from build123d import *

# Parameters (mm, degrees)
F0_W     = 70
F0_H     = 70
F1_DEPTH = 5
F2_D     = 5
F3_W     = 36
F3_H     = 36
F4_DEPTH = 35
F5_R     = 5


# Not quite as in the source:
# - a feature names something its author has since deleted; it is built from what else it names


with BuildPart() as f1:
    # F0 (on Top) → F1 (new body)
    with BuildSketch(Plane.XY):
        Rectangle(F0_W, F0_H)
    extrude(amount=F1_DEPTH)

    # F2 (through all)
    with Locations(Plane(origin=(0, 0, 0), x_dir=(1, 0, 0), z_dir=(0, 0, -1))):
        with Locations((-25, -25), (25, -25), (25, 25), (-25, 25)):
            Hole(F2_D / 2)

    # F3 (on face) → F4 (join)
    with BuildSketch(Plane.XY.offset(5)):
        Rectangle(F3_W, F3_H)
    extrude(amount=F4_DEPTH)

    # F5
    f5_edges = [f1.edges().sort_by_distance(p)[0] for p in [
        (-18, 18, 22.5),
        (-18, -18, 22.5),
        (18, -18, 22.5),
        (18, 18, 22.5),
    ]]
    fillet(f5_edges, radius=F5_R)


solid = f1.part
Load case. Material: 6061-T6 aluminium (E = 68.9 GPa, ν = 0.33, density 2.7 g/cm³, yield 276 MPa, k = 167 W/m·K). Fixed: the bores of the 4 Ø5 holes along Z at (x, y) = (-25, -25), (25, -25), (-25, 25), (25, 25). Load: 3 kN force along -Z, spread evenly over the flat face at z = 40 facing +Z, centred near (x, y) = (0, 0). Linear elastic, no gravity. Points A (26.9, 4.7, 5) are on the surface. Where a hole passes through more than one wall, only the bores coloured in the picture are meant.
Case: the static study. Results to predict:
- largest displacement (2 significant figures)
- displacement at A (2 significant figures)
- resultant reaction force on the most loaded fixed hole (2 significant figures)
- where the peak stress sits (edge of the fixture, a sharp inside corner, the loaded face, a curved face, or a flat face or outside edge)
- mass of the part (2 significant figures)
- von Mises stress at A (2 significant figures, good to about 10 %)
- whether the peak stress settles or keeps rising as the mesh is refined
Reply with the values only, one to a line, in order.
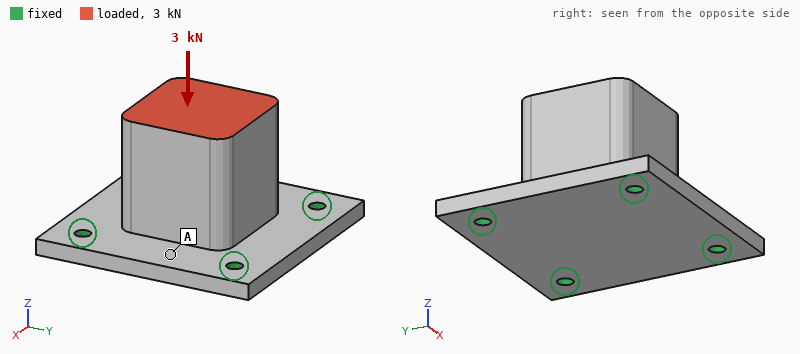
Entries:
21 µm
14 µm
800 N
edge of the fixture
190 g
11 MPa
keeps rising
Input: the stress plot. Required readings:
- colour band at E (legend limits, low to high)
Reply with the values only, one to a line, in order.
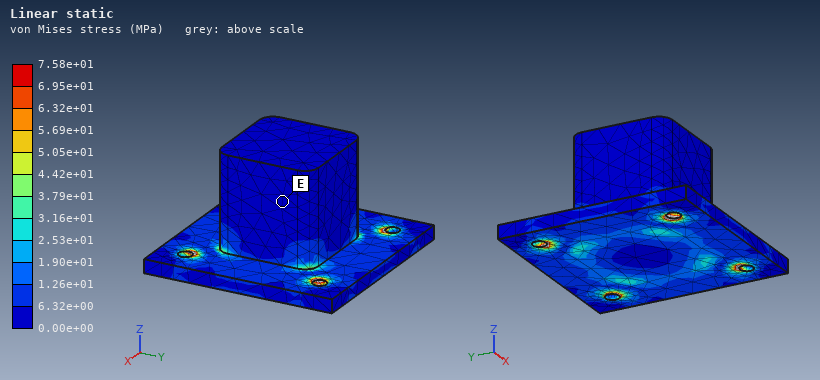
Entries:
0.00e+00 to 6.32e+00 MPa
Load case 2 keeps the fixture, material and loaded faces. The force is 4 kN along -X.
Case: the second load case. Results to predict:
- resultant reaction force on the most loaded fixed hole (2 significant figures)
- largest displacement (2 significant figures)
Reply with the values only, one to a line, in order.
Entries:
2.1 kN
0.10 mm
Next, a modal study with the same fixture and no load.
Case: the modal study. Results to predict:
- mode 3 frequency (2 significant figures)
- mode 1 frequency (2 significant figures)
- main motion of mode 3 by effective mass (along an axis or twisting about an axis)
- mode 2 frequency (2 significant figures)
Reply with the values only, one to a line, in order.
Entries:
5000 Hz
4400 Hz
along Z
4400 Hz
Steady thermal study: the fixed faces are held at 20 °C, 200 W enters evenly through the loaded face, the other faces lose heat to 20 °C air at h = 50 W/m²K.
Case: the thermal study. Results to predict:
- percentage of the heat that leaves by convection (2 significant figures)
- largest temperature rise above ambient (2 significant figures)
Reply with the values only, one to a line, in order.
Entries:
11 %
71 K
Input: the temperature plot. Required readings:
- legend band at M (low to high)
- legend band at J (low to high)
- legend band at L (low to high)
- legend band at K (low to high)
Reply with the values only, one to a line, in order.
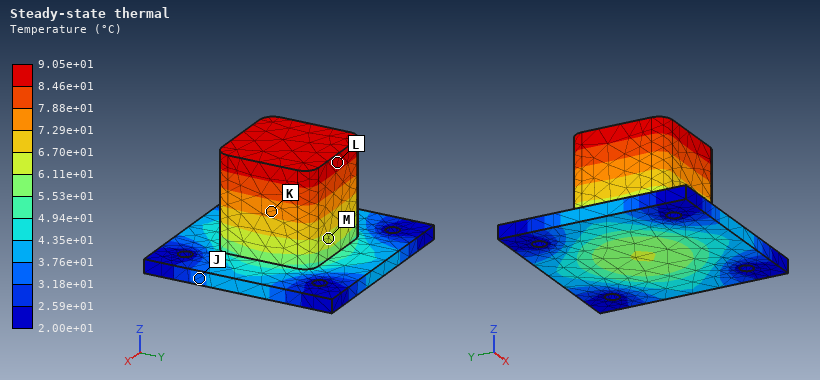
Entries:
6.11e+01 to 6.70e+01 °C
3.18e+01 to 3.76e+01 °C
8.46e+01 to 9.05e+01 °C
7.29e+01 to 7.88e+01 °C
